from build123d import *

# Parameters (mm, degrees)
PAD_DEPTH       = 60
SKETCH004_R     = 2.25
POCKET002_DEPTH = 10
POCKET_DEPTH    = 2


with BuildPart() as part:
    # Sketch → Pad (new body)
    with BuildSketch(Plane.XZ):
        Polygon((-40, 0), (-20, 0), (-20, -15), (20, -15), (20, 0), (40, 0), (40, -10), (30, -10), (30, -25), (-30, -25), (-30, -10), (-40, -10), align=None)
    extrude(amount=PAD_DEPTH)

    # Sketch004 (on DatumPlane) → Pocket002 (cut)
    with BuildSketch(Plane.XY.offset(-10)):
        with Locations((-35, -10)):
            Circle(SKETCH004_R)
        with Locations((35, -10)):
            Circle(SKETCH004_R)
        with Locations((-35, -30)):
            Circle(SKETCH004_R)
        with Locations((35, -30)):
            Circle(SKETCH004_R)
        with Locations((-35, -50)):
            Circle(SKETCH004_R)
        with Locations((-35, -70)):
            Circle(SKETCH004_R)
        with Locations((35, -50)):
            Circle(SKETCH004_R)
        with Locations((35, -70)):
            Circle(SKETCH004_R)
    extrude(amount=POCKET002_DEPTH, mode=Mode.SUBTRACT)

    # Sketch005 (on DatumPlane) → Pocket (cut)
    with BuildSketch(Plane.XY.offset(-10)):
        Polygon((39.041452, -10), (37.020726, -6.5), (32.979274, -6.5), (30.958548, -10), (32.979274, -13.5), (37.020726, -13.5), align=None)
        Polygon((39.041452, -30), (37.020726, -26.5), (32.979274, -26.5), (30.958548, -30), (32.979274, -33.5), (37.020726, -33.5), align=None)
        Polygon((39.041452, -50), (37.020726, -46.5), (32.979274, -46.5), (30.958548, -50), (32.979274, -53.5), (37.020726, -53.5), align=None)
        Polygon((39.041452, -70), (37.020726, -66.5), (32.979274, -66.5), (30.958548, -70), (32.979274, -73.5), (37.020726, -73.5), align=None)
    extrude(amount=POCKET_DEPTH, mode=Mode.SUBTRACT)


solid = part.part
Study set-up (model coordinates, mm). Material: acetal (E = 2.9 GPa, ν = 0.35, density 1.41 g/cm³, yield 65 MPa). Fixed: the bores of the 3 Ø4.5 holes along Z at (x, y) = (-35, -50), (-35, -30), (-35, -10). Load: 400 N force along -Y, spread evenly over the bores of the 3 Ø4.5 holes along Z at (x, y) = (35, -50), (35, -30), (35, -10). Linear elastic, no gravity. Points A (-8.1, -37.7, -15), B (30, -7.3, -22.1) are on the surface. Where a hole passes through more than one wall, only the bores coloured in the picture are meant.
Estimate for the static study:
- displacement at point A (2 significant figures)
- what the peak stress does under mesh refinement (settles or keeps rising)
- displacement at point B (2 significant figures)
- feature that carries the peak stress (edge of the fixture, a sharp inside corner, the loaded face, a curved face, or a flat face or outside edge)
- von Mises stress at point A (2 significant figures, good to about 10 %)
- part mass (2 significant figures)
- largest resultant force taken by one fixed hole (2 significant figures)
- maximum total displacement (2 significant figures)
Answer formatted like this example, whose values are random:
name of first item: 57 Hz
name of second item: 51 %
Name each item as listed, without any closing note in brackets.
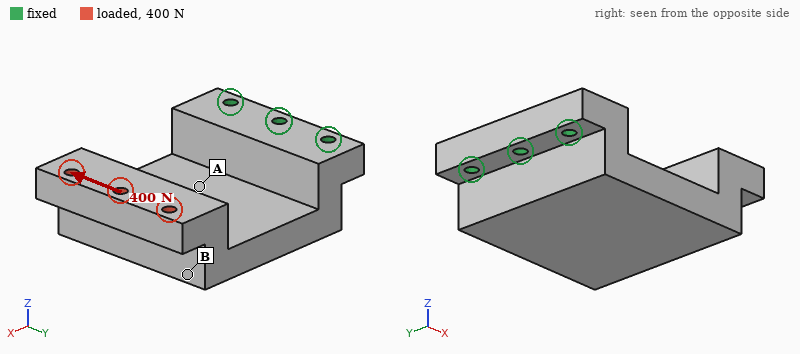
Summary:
displacement at point A: 0.18 mm
what the peak stress does under mesh refinement: keeps rising
displacement at point B: 0.59 mm
feature that carries the peak stress: edge of the fixture
von Mises stress at point A: 8.1 MPa
part mass: 91 g
largest resultant force taken by one fixed hole: 660 N
maximum total displacement: 1.0 mm
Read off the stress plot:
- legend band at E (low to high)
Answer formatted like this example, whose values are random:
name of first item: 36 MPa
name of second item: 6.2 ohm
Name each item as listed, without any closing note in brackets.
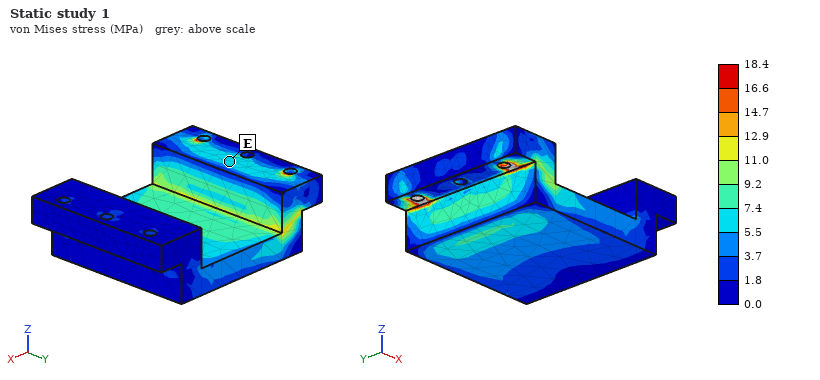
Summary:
legend band at E: 5.5 to 7.4 MPa
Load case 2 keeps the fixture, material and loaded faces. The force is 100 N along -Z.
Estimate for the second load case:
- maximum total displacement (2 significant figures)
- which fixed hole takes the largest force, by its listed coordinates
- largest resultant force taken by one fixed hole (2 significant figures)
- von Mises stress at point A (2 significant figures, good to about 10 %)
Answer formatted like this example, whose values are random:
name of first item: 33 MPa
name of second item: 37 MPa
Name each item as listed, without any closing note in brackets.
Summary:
maximum total displacement: 1.2 mm
which fixed hole takes the largest force, by its listed coordinates: (-35, -30)
largest resultant force taken by one fixed hole: 56 N
von Mises stress at point A: 4.0 MPa
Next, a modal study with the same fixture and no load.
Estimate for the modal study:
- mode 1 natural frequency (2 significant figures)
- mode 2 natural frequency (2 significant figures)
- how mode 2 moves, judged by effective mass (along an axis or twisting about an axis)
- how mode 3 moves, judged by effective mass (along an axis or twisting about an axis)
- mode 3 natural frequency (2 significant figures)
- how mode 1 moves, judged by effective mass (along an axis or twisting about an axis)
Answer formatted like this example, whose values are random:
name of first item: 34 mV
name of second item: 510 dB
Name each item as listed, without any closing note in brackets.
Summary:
mode 1 natural frequency: 300 Hz
mode 2 natural frequency: 660 Hz
how mode 2 moves, judged by effective mass: along Y
how mode 3 moves, judged by effective mass: along X
mode 3 natural frequency: 1200 Hz
how mode 1 moves, judged by effective mass: along Z
